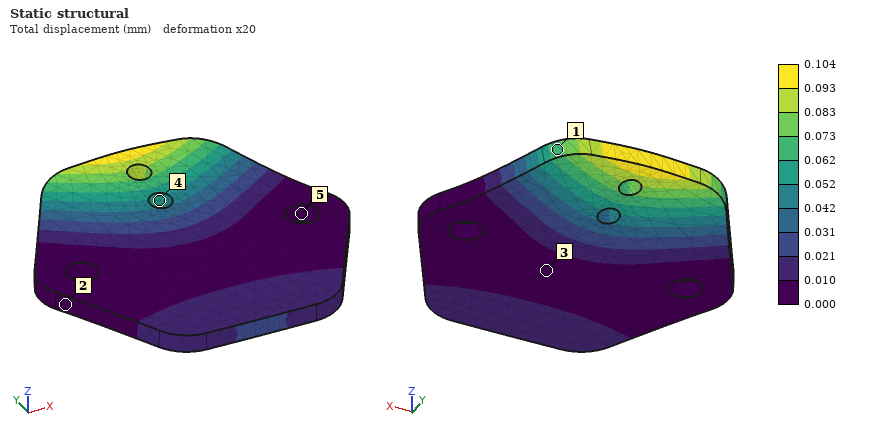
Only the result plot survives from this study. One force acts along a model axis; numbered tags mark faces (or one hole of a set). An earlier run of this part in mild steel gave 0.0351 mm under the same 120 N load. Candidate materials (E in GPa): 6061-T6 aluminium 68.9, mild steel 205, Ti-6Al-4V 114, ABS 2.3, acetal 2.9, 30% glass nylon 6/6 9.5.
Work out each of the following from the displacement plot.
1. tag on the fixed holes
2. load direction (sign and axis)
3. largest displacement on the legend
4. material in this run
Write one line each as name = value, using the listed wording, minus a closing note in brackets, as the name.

tag on the fixed holes = 5
load direction = +Z
largest displacement on the legend = 0.104 mm
material in this run = 6061-T6 aluminium
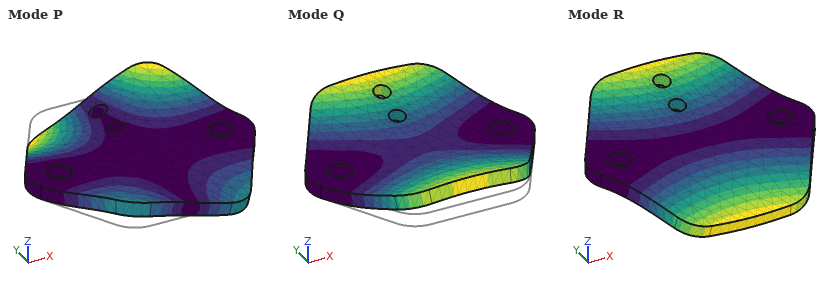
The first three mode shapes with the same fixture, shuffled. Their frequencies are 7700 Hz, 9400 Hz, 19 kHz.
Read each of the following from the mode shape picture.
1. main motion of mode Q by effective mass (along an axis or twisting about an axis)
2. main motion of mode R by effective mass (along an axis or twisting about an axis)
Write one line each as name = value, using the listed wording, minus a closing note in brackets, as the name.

main motion of mode Q by effective mass = along Z
main motion of mode R by effective mass = twisting about X
